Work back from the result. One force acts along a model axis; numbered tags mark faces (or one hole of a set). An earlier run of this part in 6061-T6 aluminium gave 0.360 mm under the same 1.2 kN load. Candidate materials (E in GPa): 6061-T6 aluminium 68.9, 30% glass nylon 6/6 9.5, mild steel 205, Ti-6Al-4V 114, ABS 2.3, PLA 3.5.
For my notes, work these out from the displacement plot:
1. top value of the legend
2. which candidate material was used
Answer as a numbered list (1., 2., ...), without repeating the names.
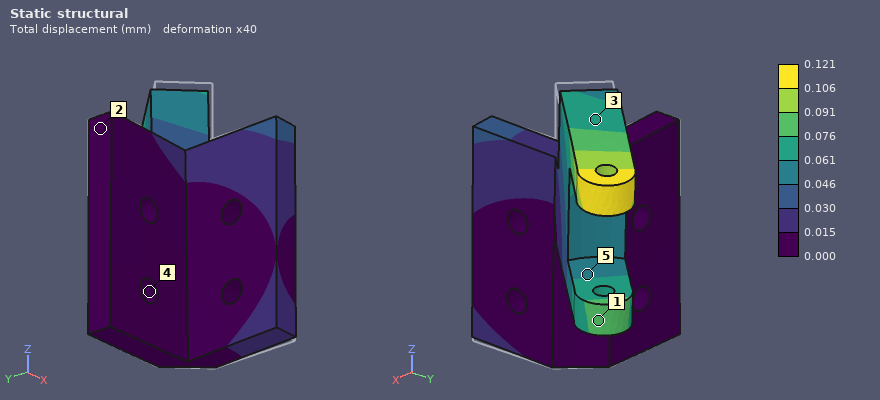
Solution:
1. 0.121 mm
2. mild steel
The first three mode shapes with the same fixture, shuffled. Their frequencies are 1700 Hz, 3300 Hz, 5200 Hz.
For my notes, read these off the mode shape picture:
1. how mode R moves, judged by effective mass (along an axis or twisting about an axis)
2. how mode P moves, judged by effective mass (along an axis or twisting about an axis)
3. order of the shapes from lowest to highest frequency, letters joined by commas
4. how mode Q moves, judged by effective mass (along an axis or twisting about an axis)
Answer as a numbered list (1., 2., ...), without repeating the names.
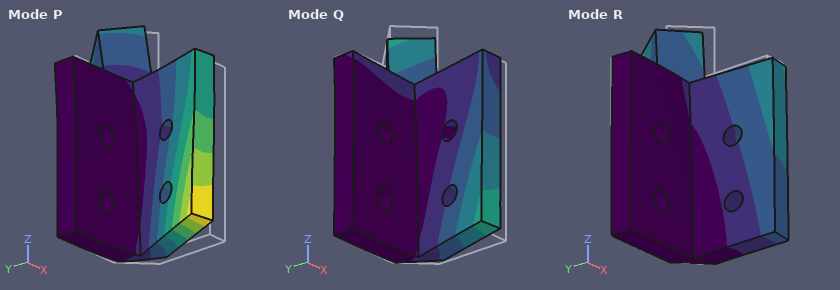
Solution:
1. along Y
2. along X
3. R, Q, P
4. along Z
